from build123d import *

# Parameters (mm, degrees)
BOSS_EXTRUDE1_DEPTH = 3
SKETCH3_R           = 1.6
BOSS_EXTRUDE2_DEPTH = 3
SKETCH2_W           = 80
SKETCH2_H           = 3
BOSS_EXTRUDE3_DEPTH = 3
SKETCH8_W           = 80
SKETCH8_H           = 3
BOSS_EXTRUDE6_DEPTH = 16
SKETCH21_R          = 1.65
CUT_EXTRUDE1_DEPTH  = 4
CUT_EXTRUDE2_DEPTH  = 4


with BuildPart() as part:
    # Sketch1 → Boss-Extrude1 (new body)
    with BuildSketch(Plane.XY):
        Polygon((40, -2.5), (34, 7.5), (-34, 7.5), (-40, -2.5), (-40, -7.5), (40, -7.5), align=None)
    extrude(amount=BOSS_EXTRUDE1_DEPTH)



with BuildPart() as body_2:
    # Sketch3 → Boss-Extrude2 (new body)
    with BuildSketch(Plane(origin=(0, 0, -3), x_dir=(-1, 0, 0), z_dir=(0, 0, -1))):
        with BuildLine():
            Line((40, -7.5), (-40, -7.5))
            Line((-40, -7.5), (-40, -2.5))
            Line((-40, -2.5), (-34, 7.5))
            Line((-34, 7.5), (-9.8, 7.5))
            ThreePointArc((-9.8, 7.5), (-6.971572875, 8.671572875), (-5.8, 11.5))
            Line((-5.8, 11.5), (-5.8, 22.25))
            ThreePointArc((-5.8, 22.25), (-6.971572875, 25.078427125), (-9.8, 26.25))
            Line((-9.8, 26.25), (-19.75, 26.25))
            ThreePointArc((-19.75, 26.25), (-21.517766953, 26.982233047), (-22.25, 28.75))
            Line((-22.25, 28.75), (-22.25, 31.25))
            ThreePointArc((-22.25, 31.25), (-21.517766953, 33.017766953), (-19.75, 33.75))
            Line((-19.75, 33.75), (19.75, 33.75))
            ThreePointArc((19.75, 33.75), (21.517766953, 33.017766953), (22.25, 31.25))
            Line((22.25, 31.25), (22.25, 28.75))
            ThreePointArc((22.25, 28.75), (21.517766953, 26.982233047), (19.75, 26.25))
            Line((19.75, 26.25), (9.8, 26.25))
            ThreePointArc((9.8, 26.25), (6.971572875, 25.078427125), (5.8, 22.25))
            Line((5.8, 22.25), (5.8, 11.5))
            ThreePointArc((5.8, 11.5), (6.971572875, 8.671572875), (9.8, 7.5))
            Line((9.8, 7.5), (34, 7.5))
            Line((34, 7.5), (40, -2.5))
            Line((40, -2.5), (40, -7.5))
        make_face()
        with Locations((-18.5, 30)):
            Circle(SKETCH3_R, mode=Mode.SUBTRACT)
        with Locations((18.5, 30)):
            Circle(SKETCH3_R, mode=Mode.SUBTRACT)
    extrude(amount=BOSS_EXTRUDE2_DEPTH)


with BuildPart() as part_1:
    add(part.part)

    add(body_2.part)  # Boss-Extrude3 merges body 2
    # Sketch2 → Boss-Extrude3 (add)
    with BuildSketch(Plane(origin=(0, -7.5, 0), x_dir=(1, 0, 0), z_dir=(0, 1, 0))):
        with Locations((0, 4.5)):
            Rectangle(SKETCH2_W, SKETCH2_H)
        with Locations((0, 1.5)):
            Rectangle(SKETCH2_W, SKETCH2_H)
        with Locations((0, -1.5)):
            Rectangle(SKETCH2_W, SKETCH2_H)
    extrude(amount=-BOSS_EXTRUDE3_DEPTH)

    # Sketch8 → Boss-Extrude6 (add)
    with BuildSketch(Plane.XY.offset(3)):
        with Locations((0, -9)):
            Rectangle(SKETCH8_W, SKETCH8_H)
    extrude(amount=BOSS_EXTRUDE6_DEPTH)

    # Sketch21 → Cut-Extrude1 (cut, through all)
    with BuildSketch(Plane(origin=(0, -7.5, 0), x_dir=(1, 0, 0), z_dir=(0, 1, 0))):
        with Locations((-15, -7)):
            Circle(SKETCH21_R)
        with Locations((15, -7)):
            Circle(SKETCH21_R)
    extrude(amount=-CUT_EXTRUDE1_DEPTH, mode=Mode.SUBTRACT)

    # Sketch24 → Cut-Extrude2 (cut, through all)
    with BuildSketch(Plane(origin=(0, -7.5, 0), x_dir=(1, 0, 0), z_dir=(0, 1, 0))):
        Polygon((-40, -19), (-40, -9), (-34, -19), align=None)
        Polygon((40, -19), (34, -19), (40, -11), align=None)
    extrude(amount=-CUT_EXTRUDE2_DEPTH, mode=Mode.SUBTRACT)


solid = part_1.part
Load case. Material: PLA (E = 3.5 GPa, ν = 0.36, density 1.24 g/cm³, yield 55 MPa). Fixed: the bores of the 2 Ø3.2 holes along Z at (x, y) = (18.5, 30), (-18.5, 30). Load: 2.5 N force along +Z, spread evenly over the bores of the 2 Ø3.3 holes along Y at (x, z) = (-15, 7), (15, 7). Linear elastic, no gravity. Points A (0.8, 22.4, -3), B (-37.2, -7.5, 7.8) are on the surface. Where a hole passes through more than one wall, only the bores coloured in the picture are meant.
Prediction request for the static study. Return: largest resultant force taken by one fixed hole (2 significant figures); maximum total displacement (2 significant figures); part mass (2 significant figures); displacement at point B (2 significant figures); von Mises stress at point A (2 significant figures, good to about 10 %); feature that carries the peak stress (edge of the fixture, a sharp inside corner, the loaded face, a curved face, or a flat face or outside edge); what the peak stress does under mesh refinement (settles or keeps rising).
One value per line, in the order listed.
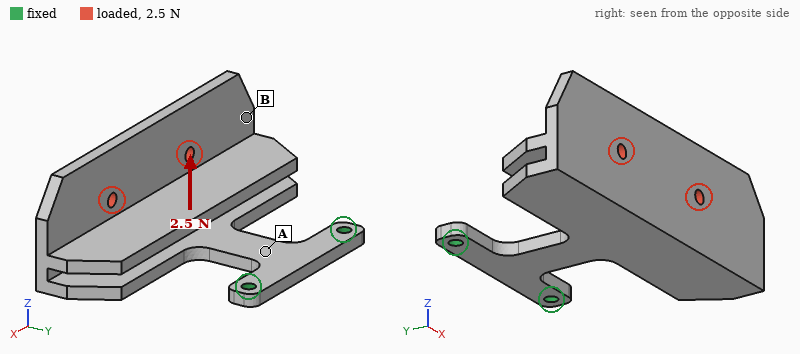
1.3 N
1.0 mm
18 g
0.80 mm
4.3 MPa
edge of the fixture
keeps rising
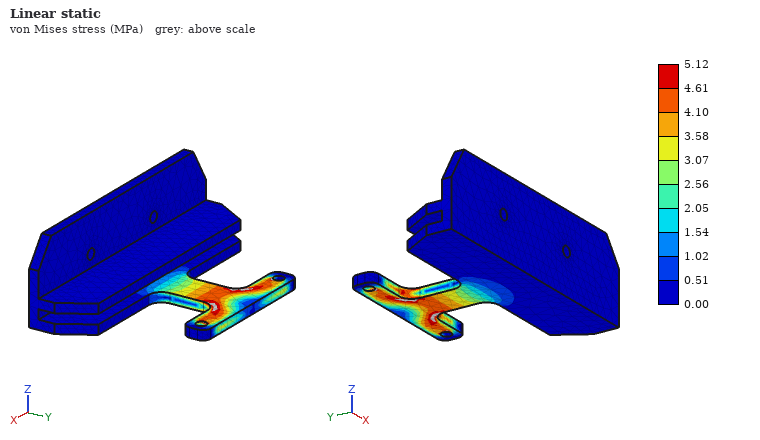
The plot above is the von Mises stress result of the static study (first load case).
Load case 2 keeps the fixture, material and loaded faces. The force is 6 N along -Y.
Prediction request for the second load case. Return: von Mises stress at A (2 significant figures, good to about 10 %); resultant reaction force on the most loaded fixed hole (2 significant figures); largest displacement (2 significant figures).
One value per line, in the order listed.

3.8 MPa
3.3 N
0.96 mm
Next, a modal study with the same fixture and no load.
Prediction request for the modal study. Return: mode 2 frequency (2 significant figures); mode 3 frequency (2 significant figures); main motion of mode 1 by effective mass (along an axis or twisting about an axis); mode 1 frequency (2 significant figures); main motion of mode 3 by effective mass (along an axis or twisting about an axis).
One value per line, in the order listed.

110 Hz
290 Hz
along Z
78 Hz
along X
